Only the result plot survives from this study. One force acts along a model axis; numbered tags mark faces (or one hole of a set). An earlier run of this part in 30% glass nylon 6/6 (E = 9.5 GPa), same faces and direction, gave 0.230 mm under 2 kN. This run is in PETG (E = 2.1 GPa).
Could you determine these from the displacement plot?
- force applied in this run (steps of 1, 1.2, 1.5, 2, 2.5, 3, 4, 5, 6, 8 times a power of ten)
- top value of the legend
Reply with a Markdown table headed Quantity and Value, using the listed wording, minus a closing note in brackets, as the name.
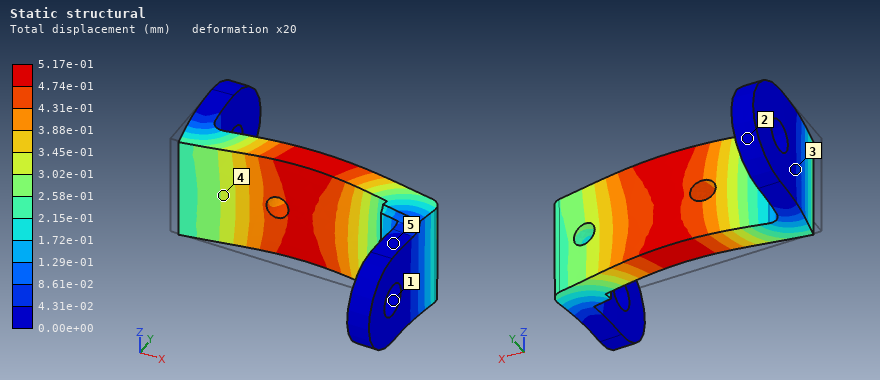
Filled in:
| Quantity | Value |
|---|---|
| force applied in this run | 1 kN |
| top value of the legend | 5.17e-01 mm |
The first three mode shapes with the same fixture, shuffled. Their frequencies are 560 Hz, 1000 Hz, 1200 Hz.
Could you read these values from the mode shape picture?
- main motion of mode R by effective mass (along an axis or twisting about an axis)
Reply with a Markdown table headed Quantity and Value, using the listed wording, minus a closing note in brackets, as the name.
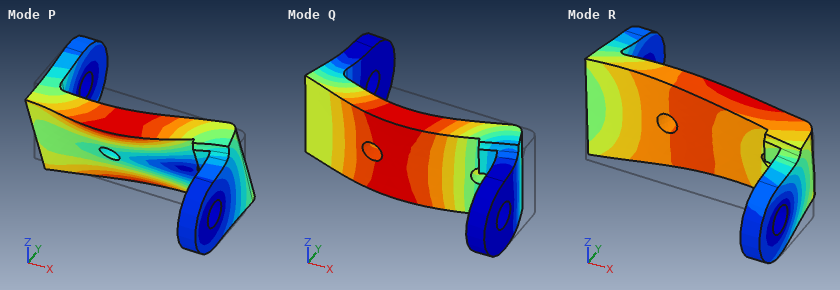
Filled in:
| Quantity | Value |
|---|---|
| main motion of mode R by effective mass | along Z |
